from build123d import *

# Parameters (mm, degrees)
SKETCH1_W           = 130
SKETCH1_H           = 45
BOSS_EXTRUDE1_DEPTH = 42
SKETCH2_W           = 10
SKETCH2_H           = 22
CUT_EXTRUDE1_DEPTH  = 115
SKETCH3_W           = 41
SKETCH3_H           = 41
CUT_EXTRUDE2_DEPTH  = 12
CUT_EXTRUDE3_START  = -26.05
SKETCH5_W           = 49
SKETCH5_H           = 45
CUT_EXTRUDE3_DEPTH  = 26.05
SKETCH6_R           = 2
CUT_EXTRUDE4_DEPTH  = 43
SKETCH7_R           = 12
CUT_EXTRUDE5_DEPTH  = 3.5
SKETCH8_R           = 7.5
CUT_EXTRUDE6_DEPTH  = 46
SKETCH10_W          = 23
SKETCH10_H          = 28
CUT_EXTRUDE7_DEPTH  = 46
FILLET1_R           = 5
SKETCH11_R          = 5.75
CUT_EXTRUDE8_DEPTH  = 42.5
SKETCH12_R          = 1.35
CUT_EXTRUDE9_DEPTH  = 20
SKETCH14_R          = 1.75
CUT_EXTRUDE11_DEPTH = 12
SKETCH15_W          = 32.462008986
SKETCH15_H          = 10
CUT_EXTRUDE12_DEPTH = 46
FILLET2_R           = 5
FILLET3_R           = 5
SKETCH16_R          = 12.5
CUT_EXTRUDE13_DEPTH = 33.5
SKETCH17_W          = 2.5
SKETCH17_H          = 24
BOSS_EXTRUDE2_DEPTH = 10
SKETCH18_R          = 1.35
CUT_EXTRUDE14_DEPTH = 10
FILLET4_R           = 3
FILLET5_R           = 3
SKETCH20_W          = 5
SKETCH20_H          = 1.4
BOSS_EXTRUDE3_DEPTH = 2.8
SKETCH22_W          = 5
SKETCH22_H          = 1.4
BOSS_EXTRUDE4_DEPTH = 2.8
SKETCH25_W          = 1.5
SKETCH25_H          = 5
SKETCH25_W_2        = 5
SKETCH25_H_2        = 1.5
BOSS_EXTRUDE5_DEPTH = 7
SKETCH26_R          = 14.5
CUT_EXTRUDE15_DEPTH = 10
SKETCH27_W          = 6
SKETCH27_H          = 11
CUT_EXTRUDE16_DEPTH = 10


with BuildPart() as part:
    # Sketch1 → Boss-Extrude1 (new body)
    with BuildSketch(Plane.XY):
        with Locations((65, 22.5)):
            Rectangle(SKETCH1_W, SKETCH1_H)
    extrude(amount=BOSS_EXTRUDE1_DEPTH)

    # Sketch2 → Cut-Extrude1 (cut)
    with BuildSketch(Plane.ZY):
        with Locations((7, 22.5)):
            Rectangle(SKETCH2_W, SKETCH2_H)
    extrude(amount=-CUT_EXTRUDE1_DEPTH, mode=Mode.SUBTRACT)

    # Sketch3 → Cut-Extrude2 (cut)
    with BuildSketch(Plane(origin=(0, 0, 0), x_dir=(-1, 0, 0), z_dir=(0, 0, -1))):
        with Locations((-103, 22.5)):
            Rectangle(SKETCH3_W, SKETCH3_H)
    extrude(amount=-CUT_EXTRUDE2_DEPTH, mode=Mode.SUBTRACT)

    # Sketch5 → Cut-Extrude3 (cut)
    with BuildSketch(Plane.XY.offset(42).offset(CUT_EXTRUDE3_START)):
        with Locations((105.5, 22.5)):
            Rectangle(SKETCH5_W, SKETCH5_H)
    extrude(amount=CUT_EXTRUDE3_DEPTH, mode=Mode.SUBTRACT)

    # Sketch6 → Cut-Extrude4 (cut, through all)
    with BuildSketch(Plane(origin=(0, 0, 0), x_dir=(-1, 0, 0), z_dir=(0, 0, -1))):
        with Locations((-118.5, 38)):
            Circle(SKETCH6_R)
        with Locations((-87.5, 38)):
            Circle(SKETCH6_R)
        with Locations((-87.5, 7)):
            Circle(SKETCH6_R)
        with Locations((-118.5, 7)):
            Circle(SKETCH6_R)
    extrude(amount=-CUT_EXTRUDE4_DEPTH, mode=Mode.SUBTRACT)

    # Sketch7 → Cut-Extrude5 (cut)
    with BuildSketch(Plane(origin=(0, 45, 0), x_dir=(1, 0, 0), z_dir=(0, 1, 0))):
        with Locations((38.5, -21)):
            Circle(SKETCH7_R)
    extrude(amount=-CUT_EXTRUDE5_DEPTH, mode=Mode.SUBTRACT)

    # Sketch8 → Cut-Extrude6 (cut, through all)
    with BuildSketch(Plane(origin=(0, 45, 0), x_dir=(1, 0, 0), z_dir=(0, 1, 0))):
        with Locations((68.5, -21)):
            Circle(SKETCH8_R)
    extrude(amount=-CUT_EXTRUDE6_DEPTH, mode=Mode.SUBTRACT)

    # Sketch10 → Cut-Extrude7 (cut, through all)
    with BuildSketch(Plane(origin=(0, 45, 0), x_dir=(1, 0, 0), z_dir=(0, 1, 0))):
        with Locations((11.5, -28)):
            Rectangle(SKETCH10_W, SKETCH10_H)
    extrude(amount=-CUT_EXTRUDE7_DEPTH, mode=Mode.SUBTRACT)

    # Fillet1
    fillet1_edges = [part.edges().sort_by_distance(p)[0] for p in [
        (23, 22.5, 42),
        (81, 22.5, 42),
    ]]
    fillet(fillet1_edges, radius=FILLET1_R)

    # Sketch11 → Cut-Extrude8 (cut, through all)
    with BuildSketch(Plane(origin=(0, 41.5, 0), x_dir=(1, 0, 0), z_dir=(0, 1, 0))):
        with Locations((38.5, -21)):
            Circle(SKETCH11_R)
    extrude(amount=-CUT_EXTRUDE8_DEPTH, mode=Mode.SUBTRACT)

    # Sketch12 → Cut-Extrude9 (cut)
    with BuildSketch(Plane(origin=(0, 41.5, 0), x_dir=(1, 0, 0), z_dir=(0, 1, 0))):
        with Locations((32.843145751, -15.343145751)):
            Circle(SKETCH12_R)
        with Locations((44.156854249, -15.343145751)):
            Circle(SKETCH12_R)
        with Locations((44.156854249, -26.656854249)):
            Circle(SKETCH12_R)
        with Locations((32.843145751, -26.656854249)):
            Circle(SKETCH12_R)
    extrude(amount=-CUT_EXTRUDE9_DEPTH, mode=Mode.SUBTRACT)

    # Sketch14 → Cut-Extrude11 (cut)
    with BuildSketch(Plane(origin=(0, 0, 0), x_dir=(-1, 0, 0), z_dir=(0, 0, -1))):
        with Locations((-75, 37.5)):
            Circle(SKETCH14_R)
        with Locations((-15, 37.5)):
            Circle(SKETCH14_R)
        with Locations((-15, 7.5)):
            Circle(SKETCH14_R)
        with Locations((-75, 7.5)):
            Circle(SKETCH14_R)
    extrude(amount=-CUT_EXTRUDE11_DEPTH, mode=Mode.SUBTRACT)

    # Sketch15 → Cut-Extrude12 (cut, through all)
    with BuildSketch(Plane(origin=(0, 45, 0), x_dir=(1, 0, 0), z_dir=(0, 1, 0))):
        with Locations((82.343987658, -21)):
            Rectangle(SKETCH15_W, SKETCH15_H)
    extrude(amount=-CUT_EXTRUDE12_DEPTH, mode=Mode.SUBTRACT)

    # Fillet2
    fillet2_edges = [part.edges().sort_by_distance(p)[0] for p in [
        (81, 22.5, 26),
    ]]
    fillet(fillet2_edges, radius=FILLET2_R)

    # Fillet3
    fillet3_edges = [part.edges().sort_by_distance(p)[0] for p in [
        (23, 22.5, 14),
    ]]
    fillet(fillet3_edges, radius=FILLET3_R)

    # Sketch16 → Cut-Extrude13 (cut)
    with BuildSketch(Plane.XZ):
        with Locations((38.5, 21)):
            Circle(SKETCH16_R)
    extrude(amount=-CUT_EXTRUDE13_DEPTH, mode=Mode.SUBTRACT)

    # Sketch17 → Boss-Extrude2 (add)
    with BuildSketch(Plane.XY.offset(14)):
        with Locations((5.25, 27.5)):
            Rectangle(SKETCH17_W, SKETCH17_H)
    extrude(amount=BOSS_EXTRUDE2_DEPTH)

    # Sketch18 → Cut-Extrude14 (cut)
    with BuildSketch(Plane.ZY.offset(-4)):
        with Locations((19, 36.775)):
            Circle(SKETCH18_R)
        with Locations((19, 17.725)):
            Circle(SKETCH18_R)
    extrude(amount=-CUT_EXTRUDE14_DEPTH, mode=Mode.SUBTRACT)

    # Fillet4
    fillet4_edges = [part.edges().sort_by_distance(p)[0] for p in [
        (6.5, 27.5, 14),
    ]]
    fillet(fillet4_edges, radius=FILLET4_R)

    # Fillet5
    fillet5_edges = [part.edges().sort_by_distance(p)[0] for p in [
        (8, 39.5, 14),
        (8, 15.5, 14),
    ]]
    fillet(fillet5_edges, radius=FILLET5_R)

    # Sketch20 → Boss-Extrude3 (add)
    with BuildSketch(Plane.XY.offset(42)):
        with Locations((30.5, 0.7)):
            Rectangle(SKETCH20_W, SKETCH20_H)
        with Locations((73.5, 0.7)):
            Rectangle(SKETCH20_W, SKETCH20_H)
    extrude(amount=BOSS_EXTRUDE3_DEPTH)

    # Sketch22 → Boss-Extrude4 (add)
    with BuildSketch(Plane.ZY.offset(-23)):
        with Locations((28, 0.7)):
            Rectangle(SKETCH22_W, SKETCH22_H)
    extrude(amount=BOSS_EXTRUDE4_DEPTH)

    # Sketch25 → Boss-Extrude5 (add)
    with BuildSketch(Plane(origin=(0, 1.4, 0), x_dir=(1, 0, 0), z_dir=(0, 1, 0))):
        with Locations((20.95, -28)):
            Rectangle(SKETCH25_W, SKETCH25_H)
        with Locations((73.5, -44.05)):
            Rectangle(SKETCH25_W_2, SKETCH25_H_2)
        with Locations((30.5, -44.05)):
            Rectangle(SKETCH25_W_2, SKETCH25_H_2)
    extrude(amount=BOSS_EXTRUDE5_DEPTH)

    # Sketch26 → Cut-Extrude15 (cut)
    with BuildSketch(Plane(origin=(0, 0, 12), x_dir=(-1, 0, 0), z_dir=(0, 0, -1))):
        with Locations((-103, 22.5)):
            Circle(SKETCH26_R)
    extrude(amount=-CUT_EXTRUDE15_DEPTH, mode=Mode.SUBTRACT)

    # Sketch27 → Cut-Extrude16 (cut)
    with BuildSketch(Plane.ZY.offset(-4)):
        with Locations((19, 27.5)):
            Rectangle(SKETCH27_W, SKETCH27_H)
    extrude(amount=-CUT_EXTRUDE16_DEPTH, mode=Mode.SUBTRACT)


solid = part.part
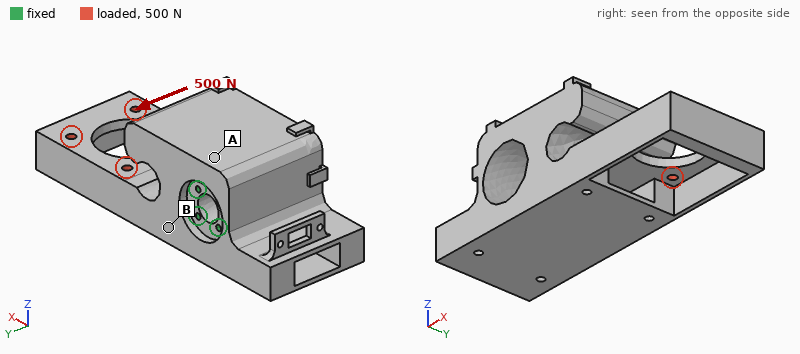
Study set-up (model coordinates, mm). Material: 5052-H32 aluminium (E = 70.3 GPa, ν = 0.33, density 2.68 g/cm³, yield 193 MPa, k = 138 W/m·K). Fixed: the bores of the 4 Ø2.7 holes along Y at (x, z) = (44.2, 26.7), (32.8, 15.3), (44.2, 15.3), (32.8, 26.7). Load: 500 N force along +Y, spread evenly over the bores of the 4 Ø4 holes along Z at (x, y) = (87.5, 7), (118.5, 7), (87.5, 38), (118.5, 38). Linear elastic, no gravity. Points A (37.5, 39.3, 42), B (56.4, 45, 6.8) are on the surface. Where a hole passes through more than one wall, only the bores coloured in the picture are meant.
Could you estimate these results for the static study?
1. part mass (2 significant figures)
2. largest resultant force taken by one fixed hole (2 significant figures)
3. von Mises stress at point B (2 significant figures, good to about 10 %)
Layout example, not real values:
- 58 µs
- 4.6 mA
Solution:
- 240 g
- 880 N
- 7.0 MPa
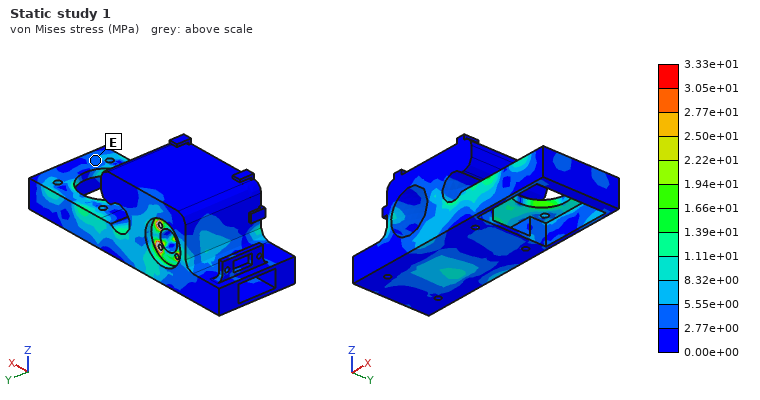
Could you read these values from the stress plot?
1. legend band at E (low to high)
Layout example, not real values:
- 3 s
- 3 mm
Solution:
- 2.77e+00 to 5.55e+00 MPa
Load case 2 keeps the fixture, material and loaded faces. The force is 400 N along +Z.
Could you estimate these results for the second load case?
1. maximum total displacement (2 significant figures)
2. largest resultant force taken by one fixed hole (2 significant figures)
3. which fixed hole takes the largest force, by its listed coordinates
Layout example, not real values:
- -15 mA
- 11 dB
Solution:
- 0.11 mm
- 1.0 kN
- (44.2, 26.7)
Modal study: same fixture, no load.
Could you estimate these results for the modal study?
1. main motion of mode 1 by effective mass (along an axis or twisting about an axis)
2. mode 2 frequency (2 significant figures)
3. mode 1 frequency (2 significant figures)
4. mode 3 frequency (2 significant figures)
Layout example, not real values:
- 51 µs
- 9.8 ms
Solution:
- along Z
- 1700 Hz
- 1600 Hz
- 2900 Hz
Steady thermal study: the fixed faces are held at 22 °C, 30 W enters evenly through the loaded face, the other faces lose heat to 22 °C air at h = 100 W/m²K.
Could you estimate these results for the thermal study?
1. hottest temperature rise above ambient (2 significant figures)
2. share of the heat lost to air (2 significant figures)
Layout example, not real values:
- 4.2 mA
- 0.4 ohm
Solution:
- 26 K
- 66 %
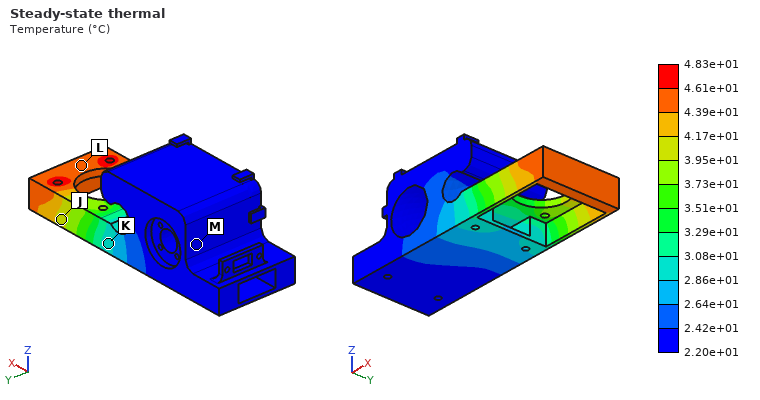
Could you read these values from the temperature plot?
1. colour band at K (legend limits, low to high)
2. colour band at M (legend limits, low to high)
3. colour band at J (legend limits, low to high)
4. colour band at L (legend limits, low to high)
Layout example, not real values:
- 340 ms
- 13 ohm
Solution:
- 2.86e+01 to 3.08e+01 °C
- 2.20e+01 to 2.42e+01 °C
- 3.95e+01 to 4.17e+01 °C
- 4.39e+01 to 4.61e+01 °C
